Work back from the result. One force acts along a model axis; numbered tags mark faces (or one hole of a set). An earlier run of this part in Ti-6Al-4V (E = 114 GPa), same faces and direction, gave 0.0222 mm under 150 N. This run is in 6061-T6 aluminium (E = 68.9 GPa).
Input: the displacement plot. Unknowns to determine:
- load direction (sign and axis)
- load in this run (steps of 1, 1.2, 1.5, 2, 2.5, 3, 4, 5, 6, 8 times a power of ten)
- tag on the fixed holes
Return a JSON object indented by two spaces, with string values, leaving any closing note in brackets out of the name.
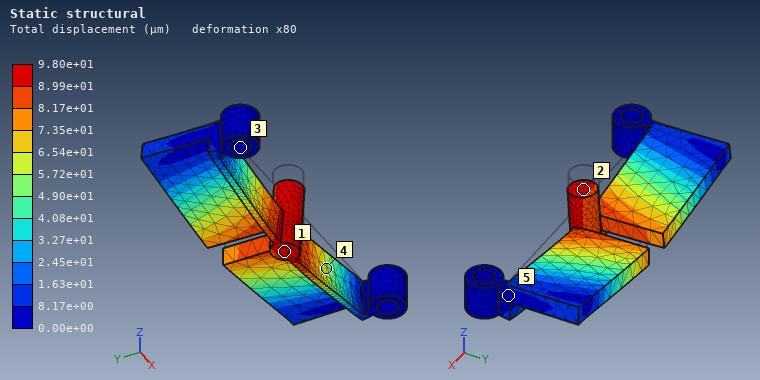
{
  "load direction": "-Z",
  "load in this run": "400 N",
  "tag on the fixed holes": "3"
}
